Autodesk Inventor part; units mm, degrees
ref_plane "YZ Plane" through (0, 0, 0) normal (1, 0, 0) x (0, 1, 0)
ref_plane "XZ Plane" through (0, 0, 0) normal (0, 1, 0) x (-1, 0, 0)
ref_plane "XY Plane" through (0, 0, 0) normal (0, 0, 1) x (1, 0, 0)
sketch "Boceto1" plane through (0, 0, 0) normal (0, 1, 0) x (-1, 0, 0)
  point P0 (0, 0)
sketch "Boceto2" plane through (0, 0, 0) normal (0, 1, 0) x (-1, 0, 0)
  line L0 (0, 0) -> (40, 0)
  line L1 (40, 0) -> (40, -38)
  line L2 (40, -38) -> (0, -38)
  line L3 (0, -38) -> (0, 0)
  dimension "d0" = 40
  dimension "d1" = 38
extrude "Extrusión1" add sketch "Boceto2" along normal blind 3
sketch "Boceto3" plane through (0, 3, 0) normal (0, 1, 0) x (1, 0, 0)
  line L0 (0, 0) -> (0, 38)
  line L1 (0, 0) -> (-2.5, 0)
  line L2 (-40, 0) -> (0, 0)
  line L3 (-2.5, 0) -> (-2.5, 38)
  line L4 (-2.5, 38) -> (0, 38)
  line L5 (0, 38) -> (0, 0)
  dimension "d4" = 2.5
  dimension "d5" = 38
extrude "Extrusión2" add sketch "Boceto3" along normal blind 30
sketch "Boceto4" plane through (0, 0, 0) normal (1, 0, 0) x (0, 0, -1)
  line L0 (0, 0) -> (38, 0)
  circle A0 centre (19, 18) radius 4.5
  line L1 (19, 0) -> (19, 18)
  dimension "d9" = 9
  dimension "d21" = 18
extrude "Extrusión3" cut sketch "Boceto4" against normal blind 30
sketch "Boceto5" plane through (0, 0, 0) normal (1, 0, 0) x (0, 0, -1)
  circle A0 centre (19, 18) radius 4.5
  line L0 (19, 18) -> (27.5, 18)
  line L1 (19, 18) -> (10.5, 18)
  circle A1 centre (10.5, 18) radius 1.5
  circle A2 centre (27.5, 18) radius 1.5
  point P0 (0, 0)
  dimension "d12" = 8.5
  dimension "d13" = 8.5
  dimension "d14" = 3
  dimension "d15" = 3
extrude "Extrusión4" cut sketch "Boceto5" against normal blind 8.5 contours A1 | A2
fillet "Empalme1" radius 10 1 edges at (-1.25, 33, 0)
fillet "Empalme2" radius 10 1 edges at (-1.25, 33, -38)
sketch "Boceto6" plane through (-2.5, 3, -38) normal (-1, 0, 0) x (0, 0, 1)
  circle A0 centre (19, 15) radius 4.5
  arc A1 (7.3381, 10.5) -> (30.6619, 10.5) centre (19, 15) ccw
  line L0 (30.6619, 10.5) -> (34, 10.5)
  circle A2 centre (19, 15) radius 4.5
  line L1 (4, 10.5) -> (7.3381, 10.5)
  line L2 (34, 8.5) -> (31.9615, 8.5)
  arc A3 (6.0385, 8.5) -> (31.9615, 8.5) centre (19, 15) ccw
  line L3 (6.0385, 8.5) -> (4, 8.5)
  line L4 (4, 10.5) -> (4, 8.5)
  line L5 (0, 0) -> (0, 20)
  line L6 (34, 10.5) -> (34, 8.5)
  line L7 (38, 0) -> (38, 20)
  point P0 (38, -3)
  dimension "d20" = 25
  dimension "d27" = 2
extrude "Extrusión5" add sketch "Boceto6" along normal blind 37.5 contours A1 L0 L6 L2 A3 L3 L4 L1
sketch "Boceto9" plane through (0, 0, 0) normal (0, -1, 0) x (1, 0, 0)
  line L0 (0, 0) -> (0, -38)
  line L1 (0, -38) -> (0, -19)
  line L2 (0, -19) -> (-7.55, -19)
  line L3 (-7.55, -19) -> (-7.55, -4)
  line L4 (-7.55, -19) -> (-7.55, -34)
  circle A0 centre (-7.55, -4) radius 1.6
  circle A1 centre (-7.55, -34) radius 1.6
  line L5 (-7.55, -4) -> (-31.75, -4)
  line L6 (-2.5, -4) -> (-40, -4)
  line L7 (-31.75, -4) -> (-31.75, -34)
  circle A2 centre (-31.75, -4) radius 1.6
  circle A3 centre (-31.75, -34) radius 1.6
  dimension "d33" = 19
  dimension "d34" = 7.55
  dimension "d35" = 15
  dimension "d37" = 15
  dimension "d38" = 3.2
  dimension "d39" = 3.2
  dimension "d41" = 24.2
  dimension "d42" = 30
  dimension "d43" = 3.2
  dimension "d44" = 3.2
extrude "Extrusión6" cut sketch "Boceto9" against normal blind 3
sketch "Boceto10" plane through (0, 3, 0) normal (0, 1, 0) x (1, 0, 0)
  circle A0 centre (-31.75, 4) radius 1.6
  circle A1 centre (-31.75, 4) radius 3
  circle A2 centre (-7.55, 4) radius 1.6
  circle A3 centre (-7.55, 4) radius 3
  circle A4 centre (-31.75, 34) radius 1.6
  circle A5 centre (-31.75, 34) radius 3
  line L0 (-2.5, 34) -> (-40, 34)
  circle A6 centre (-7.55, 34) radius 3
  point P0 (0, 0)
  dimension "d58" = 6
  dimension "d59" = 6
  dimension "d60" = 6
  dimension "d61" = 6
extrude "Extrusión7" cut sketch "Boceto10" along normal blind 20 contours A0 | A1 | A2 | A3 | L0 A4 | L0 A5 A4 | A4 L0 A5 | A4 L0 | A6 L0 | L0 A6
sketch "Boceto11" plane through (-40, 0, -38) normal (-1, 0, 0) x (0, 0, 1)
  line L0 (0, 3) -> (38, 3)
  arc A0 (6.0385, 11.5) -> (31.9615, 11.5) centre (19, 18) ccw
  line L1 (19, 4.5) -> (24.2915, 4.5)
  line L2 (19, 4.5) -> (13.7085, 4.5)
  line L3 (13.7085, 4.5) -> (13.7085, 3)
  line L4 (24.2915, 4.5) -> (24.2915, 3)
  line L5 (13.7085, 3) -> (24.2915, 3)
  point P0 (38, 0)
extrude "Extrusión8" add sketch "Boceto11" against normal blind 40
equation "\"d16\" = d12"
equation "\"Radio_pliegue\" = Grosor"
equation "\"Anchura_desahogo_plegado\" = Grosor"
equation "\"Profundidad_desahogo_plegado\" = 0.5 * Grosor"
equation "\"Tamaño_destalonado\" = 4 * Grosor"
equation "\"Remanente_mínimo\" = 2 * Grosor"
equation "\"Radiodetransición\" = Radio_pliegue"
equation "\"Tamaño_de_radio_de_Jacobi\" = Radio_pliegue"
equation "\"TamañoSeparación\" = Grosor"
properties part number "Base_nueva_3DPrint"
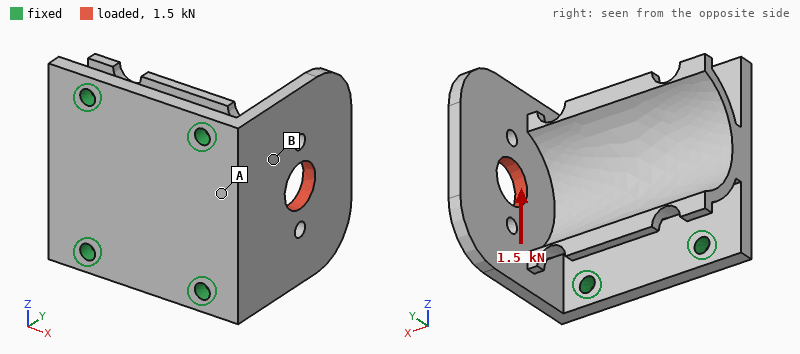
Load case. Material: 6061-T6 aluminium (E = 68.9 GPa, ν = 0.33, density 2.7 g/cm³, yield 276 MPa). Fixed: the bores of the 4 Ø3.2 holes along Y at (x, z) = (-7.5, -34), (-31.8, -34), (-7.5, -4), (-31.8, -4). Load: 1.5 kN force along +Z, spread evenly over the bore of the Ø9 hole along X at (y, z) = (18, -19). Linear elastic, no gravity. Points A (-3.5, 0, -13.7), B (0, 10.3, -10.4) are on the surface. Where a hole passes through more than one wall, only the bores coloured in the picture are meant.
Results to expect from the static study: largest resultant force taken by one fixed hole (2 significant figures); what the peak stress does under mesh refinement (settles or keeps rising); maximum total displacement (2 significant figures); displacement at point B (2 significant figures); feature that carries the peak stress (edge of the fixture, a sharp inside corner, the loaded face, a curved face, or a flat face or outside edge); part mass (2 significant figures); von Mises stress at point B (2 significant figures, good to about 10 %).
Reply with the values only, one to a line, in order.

1.1 kN
keeps rising
65 µm
21 µm
edge of the fixture
27 g
33 MPa
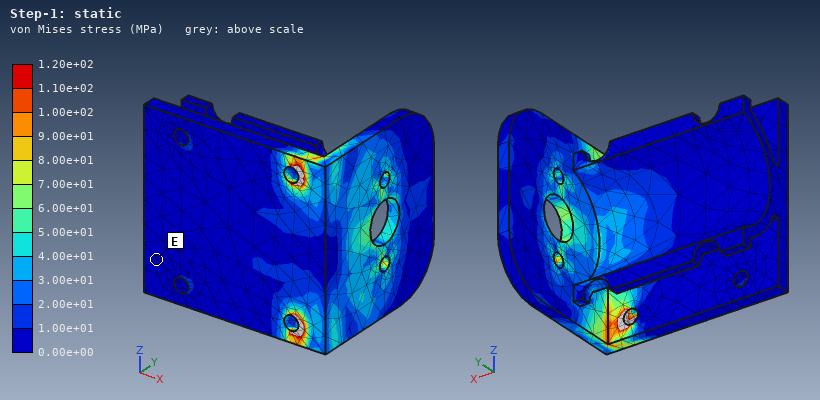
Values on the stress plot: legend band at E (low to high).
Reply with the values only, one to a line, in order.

0.00e+00 to 1.00e+01 MPa
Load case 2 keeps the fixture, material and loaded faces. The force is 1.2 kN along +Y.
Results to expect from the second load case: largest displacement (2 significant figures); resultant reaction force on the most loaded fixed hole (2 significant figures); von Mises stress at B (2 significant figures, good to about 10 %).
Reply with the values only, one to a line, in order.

30 µm
690 N
18 MPa
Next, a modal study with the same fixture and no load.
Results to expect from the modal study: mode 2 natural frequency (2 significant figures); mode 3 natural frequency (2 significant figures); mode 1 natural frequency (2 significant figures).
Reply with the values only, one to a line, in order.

7200 Hz
8900 Hz
3500 Hz
